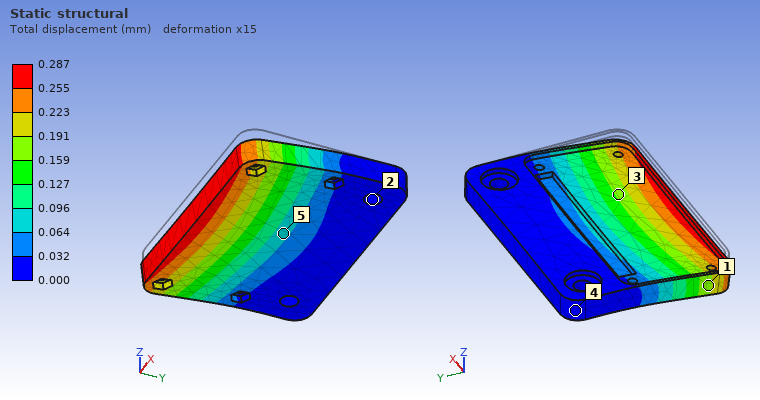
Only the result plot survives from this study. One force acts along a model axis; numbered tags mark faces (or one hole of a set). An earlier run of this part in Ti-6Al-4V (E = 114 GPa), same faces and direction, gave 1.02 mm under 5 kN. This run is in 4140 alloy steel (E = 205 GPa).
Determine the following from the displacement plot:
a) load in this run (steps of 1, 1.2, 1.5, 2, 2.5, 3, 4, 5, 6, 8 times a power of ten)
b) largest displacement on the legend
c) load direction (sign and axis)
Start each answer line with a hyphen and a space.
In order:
- 2.5 kN
- 0.287 mm
- -Z
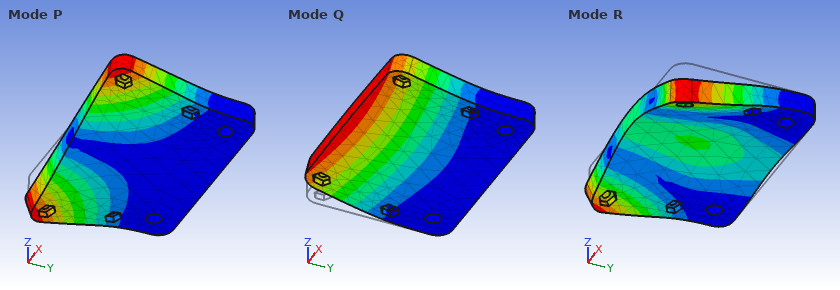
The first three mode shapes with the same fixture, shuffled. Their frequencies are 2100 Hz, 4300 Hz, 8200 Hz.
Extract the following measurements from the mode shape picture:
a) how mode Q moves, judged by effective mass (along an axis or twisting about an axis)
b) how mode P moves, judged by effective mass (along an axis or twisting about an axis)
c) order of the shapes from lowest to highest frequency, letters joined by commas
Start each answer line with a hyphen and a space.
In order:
- along Z
- twisting about Y
- Q, P, R
